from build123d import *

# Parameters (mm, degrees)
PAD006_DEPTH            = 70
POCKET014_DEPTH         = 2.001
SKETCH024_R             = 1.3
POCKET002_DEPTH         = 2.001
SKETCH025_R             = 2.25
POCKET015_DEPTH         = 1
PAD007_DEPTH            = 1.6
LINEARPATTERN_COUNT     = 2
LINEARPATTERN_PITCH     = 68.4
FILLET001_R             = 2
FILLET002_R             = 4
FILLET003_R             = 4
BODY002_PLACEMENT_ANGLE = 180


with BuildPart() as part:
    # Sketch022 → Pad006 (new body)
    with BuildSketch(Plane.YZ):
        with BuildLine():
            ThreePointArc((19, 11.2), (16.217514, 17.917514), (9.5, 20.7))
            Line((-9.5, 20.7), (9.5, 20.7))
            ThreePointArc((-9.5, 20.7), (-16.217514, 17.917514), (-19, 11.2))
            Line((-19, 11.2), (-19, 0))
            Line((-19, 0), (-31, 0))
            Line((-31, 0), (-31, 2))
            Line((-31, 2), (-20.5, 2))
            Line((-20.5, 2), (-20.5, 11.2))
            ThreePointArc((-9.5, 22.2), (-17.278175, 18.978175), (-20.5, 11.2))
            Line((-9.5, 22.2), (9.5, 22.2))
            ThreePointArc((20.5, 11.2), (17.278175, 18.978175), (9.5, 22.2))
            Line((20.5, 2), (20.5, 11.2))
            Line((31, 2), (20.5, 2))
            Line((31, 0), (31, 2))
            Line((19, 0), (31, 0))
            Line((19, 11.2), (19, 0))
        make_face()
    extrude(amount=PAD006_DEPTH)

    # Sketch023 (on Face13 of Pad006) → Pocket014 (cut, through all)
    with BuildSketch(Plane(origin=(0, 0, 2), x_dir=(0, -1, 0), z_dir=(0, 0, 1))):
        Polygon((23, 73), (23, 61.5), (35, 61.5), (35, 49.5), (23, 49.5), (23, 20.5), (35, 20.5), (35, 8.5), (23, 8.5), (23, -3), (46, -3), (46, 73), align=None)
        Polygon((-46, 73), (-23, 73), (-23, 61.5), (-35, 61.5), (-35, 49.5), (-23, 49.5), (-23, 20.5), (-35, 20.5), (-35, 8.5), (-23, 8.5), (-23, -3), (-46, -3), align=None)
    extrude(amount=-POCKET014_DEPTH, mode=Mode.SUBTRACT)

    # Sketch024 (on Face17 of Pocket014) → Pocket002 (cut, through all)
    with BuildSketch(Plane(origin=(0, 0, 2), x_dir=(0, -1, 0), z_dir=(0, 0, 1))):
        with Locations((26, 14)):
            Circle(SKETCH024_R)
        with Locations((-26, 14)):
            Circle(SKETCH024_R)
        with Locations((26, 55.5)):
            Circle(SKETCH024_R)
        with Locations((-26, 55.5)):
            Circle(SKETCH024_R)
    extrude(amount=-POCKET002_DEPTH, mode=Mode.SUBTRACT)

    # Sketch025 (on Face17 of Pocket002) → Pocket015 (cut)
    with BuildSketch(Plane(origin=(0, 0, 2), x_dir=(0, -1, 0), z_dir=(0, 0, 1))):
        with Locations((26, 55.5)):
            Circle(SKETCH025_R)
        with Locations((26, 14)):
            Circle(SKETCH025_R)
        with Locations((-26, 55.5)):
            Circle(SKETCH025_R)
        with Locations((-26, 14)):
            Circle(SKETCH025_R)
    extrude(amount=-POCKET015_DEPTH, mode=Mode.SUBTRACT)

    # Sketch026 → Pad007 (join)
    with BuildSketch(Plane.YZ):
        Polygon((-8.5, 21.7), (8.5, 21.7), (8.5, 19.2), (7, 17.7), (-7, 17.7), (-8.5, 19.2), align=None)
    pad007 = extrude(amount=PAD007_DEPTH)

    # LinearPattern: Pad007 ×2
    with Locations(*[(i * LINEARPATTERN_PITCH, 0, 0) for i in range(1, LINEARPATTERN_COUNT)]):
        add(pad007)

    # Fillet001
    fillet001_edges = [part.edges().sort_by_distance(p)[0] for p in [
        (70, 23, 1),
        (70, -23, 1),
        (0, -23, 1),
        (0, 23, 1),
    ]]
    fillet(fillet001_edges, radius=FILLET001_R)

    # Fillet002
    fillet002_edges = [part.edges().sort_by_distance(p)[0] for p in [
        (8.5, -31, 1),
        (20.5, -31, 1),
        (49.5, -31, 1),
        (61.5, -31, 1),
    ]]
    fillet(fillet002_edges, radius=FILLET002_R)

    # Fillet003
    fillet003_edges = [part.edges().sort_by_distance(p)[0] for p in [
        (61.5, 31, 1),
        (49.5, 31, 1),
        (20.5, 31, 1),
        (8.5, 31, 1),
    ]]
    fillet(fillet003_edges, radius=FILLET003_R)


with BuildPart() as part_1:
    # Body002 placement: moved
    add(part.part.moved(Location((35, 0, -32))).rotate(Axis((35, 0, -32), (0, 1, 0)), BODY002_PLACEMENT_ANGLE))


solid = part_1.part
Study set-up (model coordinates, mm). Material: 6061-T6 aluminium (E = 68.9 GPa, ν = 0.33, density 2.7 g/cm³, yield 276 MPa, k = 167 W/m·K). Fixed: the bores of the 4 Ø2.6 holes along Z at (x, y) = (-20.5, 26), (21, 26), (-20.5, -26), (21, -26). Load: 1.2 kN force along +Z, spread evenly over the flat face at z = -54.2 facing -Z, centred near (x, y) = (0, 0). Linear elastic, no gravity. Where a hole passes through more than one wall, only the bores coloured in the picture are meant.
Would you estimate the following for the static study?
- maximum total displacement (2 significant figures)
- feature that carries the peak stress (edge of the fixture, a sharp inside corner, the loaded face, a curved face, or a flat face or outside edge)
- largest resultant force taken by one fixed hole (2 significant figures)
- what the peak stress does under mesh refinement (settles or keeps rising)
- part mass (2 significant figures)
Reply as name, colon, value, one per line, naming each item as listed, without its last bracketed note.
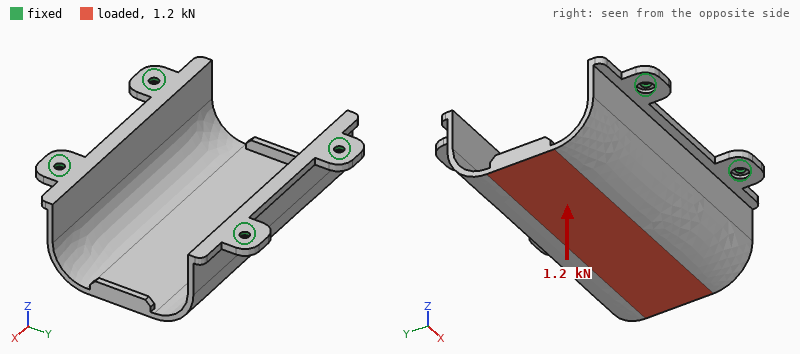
maximum total displacement: 0.22 mm
feature that carries the peak stress: edge of the fixture
largest resultant force taken by one fixed hole: 360 N
what the peak stress does under mesh refinement: keeps rising
part mass: 25 g
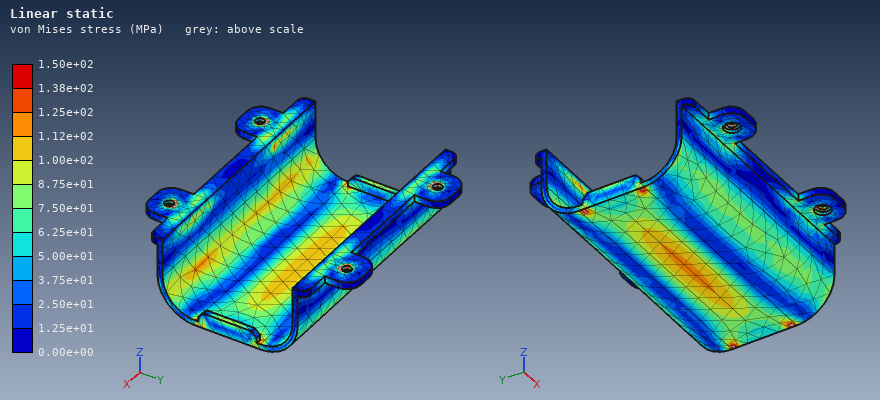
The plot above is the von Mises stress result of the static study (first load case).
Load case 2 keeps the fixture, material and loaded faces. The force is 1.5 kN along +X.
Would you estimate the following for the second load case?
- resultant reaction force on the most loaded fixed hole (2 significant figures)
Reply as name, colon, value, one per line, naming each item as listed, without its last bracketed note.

resultant reaction force on the most loaded fixed hole: 560 N
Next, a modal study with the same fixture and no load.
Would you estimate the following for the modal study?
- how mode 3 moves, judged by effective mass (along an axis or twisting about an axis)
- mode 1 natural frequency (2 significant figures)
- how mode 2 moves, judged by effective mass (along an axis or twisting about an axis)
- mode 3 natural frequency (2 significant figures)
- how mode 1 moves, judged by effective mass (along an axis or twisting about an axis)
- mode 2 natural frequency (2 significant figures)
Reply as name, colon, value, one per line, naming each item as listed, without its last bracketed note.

how mode 3 moves, judged by effective mass: along X
mode 1 natural frequency: 1900 Hz
how mode 2 moves, judged by effective mass: twisting about Z
mode 3 natural frequency: 4200 Hz
how mode 1 moves, judged by effective mass: along Y
mode 2 natural frequency: 3500 Hz
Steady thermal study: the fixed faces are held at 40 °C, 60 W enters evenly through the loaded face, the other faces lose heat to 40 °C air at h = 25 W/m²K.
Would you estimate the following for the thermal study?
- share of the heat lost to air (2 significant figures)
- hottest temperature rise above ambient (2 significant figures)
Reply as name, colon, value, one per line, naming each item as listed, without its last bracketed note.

share of the heat lost to air: 21 %
hottest temperature rise above ambient: 75 K
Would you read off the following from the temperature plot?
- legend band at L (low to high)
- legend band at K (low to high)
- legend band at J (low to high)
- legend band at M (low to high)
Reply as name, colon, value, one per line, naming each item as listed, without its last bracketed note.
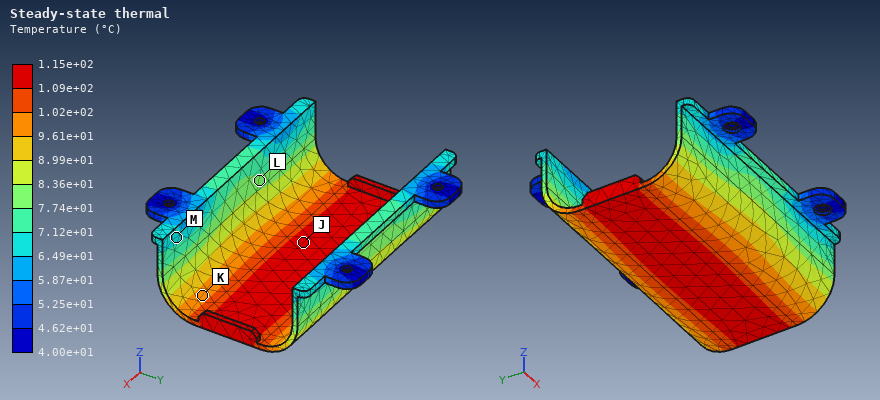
legend band at L: 7.74e+01 to 8.36e+01 °C
legend band at K: 9.61e+01 to 1.02e+02 °C
legend band at J: 1.09e+02 to 1.15e+02 °C
legend band at M: 6.49e+01 to 7.12e+01 °C
